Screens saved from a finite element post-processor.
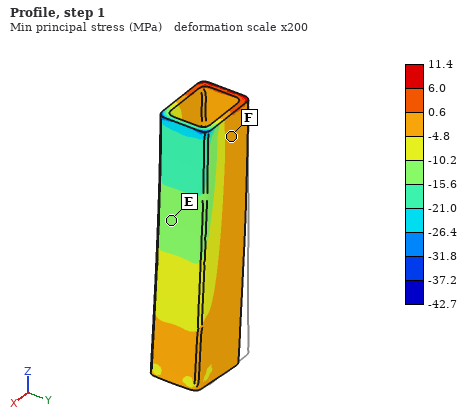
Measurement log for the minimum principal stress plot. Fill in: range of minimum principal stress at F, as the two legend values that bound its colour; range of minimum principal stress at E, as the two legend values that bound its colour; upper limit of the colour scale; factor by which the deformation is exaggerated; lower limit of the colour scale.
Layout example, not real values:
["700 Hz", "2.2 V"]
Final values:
["-4.8 to 0.6 MPa", "-15.6 to -10.2 MPa", "11.4 MPa", "200", "-42.7 MPa"]
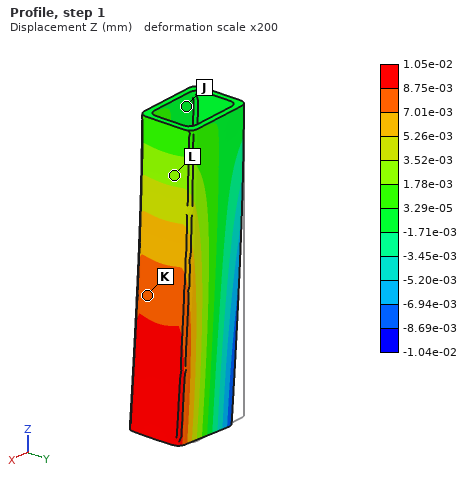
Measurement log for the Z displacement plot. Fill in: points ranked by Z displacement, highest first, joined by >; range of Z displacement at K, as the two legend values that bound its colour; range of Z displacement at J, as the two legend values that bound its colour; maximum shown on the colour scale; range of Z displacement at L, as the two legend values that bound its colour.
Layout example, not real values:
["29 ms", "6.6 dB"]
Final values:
["K > L > J", "7.01e-03 to 8.75e-03 mm", "-1.71e-03 to 3.29e-05 mm", "1.05e-02 mm", "1.78e-03 to 3.52e-03 mm"]
